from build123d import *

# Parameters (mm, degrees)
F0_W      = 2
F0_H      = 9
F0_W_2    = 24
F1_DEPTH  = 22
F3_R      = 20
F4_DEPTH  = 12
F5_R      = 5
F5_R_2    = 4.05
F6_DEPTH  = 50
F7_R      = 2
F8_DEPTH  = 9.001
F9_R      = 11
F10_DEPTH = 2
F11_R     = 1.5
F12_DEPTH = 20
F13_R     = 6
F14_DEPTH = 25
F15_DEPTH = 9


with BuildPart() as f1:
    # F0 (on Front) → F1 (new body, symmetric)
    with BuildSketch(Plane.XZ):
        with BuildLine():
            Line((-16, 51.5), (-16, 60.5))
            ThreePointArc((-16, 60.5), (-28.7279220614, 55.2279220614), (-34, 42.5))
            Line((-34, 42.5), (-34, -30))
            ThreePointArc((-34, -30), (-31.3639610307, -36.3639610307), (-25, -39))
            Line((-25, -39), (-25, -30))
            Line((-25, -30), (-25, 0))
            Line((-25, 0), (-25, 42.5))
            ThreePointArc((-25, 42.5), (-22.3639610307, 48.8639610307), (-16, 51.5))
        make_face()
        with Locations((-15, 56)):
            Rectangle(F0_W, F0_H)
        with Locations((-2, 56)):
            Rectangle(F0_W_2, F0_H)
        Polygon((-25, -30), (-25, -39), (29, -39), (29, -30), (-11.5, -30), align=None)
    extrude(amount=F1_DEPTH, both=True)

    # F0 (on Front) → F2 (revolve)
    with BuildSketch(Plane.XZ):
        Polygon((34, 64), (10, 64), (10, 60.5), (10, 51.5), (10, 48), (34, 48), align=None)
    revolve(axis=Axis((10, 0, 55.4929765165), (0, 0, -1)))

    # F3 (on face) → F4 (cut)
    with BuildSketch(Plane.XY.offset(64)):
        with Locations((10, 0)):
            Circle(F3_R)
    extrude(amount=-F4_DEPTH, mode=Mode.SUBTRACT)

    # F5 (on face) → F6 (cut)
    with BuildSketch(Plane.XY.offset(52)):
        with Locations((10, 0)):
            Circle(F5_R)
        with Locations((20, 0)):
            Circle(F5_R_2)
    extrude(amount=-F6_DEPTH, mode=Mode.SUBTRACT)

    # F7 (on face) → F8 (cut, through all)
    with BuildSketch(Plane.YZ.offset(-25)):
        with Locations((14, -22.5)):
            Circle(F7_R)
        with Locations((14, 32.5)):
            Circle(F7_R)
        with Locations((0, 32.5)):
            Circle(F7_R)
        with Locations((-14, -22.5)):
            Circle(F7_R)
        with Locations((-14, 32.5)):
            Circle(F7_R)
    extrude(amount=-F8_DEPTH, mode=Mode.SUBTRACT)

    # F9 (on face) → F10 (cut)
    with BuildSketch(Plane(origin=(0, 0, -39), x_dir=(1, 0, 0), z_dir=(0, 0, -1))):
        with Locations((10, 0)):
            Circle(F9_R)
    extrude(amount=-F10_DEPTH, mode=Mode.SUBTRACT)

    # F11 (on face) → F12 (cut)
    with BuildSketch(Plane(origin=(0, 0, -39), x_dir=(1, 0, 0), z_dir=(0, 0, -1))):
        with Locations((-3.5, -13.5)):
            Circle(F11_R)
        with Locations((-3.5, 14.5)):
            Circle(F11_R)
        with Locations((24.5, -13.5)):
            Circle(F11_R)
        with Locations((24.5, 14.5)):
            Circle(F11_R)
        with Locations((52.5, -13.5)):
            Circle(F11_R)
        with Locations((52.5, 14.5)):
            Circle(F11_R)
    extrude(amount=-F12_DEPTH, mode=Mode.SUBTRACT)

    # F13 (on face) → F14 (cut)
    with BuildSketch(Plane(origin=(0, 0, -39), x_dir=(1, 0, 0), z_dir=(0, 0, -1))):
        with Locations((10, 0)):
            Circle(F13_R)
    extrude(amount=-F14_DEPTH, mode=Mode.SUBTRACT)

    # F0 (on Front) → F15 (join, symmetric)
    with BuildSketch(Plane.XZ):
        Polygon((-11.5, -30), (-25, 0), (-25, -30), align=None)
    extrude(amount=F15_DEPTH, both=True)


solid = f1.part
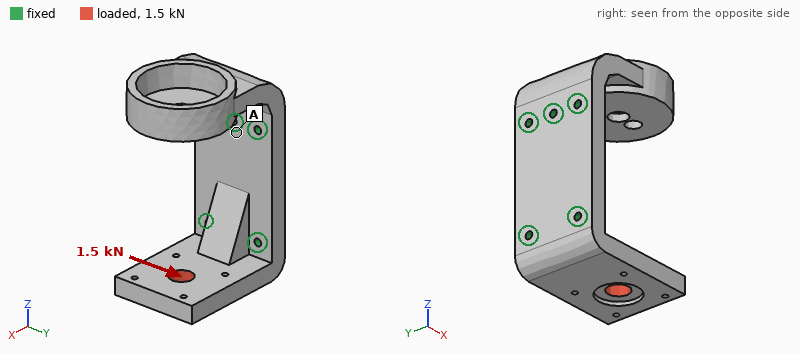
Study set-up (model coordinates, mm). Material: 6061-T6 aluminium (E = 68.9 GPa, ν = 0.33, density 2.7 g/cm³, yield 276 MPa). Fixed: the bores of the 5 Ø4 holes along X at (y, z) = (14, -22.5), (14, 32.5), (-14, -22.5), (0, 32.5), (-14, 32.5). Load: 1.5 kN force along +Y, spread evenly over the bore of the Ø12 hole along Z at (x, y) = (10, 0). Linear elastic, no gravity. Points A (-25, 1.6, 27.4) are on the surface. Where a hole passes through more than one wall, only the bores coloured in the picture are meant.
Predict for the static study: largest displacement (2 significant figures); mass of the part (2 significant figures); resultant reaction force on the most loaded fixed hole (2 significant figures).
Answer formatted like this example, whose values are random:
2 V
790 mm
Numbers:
51 µm
210 g
2.1 kN
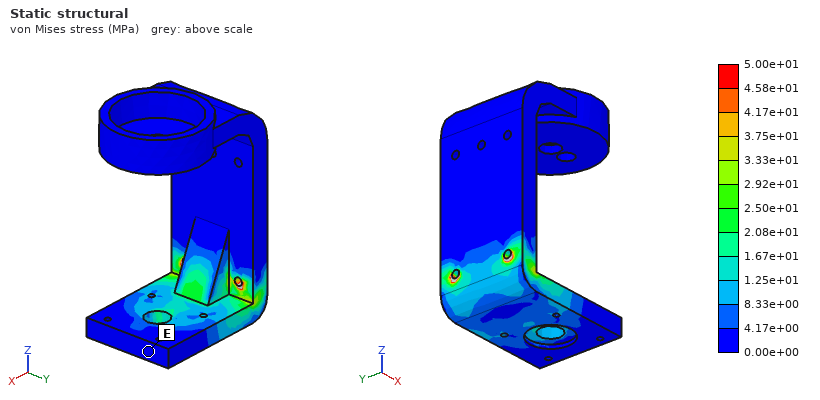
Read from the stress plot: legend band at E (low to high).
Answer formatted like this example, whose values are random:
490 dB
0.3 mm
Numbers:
0.00e+00 to 4.17e+00 MPa
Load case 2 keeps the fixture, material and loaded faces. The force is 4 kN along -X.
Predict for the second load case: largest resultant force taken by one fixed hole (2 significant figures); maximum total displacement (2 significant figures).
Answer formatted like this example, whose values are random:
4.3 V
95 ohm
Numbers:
2.2 kN
45 µm
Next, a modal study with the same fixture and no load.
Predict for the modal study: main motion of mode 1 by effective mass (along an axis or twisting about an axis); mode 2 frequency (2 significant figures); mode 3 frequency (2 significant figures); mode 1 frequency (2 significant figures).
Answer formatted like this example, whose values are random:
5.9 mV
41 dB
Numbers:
along Z
2600 Hz
2600 Hz
1400 Hz
